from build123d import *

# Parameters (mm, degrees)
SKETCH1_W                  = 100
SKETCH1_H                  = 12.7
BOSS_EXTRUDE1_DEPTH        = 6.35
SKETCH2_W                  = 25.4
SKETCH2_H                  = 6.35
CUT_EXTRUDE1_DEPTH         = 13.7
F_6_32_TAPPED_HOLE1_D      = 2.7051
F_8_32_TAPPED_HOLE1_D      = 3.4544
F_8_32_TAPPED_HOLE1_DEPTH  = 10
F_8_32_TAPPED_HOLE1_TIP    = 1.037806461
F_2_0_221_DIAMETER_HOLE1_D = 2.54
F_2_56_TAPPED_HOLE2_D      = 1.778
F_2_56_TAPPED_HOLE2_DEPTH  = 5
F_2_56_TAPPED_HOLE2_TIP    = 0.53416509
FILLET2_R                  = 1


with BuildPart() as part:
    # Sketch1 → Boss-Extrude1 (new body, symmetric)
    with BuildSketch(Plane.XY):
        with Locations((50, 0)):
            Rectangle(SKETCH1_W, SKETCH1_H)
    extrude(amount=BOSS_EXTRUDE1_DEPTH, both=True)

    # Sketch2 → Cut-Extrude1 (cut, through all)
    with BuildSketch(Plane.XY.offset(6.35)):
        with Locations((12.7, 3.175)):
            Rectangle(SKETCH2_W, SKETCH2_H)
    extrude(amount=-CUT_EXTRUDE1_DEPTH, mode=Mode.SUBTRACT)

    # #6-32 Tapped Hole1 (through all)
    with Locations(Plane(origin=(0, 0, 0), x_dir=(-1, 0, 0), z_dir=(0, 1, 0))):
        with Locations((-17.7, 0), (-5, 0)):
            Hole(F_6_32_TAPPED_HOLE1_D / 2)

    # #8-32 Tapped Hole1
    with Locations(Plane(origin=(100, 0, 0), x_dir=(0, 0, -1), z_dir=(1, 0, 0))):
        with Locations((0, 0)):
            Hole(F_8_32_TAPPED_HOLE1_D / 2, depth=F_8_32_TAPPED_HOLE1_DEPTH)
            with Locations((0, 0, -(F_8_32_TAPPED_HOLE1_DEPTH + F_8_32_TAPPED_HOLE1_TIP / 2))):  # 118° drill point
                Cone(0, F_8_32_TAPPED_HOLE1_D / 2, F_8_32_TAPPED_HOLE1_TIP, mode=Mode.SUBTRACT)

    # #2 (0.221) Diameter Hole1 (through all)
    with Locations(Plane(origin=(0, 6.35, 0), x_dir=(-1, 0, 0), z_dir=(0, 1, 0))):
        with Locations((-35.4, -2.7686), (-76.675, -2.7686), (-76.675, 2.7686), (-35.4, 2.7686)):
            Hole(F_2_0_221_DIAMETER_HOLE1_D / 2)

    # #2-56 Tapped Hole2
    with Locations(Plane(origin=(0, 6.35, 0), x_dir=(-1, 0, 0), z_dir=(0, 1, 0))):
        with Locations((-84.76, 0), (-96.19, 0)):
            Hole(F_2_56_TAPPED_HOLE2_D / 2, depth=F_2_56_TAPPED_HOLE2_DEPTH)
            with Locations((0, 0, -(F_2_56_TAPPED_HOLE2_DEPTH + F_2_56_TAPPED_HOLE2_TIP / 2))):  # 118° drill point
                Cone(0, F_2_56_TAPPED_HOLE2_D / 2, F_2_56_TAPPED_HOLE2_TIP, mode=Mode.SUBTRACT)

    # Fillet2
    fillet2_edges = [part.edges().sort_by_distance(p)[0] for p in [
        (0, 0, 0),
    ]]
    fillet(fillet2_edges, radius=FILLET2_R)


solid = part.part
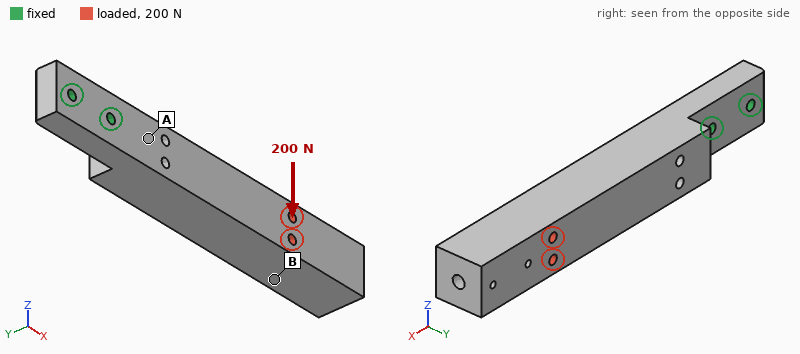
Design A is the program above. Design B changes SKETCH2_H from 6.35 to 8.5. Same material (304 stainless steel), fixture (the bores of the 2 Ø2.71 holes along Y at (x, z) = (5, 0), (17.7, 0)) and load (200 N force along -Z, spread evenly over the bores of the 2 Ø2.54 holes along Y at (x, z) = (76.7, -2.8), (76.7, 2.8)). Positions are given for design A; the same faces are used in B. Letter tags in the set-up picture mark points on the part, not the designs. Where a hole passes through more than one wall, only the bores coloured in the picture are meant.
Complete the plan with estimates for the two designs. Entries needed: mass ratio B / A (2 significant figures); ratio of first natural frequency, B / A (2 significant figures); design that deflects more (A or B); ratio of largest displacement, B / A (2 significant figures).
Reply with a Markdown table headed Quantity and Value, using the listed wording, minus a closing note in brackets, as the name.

| Quantity | Value |
|---|---|
| mass ratio B / A | 0.98 |
| ratio of first natural frequency, B / A | 0.80 |
| design that deflects more | B |
| ratio of largest displacement, B / A | 1.1 |
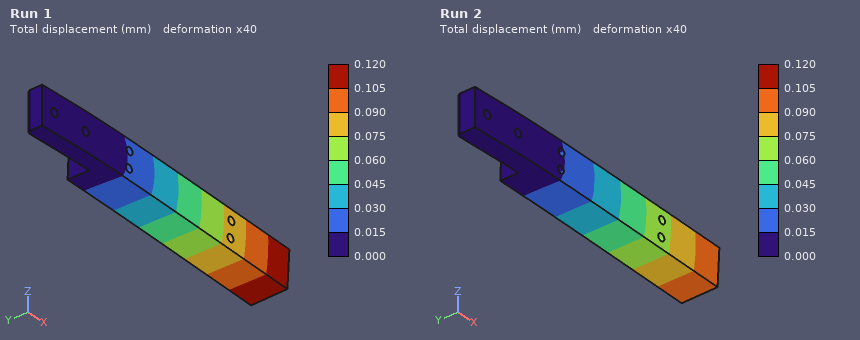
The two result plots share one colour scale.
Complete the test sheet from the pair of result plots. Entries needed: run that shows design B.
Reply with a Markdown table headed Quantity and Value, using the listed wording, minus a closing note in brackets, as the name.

| Quantity | Value |
|---|---|
| run that shows design B | Run 1 |
